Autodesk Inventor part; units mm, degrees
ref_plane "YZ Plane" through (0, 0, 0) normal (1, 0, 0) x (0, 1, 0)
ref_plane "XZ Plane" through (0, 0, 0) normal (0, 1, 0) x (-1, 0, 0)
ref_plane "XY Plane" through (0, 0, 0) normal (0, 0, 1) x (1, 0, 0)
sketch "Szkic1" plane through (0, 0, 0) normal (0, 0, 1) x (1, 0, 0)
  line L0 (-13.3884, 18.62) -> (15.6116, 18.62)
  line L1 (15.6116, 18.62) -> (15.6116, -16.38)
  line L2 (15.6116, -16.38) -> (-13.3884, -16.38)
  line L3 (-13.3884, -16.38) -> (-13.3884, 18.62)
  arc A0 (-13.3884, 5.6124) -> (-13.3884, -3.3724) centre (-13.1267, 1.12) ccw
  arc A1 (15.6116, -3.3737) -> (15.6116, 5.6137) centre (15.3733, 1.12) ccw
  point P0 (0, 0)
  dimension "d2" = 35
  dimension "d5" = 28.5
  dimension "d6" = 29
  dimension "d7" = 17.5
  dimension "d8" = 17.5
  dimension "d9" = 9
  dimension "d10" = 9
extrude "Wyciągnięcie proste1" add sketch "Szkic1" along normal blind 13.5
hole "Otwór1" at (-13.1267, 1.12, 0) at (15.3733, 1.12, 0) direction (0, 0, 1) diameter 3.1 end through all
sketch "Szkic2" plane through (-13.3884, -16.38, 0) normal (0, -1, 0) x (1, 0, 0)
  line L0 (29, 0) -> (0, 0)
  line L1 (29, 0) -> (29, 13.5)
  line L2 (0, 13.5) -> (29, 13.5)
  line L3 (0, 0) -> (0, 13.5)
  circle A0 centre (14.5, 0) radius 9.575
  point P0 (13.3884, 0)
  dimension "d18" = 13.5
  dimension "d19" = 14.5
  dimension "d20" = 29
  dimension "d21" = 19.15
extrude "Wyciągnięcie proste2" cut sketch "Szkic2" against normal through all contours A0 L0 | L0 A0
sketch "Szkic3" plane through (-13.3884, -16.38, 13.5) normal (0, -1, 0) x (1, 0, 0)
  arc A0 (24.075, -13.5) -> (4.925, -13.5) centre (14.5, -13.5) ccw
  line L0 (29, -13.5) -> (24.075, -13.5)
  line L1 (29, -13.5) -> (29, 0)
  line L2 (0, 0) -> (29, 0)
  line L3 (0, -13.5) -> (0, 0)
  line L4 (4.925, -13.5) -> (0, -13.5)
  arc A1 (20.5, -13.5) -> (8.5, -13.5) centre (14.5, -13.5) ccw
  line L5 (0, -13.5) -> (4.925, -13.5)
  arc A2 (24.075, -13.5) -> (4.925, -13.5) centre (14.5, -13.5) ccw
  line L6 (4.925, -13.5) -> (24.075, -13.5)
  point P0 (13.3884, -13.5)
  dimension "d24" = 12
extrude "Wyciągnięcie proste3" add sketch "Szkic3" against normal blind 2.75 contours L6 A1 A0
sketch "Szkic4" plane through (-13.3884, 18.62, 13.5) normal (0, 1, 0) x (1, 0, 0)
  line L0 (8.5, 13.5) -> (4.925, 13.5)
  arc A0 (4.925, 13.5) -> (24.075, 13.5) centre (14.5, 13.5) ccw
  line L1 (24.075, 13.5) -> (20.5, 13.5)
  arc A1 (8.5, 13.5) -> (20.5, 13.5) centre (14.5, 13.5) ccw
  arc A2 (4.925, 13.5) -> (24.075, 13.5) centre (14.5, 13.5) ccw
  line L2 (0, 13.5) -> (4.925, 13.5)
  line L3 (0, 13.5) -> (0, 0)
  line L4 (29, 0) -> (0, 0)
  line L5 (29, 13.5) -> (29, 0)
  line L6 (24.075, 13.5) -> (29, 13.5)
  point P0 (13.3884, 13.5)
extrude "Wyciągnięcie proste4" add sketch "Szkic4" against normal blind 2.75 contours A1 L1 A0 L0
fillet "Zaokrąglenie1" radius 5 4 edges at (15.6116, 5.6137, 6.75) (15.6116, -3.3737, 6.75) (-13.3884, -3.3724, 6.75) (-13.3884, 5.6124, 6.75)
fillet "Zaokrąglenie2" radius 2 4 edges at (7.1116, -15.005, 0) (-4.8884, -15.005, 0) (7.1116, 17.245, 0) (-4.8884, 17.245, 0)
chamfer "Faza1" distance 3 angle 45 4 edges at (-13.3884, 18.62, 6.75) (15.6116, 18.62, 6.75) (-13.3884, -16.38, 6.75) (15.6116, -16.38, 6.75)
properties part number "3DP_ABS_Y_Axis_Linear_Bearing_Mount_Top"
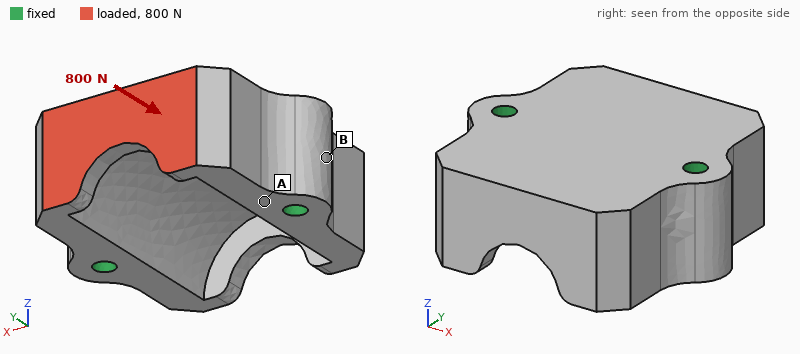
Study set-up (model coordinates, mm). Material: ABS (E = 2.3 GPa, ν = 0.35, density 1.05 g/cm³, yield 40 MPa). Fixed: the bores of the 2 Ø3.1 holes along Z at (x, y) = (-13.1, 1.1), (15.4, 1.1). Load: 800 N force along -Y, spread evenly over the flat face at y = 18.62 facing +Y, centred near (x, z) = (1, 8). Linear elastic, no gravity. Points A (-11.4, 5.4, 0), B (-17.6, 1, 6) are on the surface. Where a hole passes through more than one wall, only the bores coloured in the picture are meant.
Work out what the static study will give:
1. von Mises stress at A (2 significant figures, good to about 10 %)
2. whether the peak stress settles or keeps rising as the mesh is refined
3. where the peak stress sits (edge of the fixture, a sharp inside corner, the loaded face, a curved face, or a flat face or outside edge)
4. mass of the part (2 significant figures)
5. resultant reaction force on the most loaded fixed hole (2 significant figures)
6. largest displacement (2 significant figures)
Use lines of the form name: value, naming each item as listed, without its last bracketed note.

von Mises stress at A: 4.1 MPa
whether the peak stress settles or keeps rising as the mesh is refined: keeps rising
where the peak stress sits: a sharp inside corner
mass of the part: 10 g
resultant reaction force on the most loaded fixed hole: 410 N
largest displacement: 0.11 mm
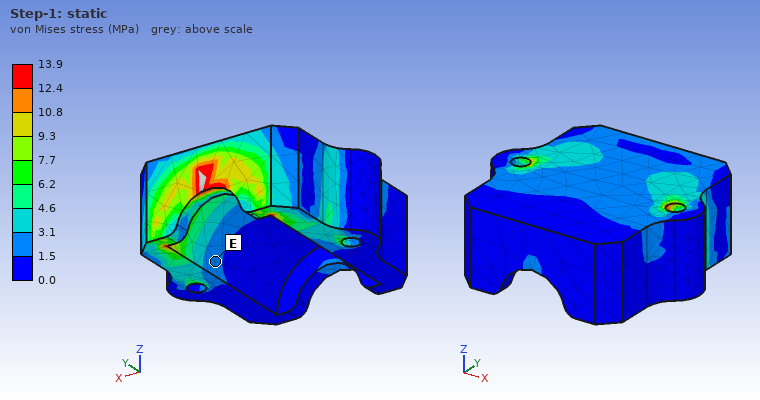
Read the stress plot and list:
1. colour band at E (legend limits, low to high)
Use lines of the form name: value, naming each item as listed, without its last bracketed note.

colour band at E: 1.5 to 3.1 MPa
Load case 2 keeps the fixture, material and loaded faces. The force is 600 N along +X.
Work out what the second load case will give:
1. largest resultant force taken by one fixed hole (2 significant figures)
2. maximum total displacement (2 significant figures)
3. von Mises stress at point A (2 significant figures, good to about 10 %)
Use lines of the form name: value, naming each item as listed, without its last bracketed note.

largest resultant force taken by one fixed hole: 450 N
maximum total displacement: 0.19 mm
von Mises stress at point A: 3.4 MPa
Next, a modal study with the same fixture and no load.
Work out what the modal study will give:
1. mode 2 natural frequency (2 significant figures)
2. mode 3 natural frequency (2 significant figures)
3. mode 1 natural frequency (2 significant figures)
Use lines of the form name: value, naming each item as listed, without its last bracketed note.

mode 2 natural frequency: 7100 Hz
mode 3 natural frequency: 7300 Hz
mode 1 natural frequency: 5900 Hz
